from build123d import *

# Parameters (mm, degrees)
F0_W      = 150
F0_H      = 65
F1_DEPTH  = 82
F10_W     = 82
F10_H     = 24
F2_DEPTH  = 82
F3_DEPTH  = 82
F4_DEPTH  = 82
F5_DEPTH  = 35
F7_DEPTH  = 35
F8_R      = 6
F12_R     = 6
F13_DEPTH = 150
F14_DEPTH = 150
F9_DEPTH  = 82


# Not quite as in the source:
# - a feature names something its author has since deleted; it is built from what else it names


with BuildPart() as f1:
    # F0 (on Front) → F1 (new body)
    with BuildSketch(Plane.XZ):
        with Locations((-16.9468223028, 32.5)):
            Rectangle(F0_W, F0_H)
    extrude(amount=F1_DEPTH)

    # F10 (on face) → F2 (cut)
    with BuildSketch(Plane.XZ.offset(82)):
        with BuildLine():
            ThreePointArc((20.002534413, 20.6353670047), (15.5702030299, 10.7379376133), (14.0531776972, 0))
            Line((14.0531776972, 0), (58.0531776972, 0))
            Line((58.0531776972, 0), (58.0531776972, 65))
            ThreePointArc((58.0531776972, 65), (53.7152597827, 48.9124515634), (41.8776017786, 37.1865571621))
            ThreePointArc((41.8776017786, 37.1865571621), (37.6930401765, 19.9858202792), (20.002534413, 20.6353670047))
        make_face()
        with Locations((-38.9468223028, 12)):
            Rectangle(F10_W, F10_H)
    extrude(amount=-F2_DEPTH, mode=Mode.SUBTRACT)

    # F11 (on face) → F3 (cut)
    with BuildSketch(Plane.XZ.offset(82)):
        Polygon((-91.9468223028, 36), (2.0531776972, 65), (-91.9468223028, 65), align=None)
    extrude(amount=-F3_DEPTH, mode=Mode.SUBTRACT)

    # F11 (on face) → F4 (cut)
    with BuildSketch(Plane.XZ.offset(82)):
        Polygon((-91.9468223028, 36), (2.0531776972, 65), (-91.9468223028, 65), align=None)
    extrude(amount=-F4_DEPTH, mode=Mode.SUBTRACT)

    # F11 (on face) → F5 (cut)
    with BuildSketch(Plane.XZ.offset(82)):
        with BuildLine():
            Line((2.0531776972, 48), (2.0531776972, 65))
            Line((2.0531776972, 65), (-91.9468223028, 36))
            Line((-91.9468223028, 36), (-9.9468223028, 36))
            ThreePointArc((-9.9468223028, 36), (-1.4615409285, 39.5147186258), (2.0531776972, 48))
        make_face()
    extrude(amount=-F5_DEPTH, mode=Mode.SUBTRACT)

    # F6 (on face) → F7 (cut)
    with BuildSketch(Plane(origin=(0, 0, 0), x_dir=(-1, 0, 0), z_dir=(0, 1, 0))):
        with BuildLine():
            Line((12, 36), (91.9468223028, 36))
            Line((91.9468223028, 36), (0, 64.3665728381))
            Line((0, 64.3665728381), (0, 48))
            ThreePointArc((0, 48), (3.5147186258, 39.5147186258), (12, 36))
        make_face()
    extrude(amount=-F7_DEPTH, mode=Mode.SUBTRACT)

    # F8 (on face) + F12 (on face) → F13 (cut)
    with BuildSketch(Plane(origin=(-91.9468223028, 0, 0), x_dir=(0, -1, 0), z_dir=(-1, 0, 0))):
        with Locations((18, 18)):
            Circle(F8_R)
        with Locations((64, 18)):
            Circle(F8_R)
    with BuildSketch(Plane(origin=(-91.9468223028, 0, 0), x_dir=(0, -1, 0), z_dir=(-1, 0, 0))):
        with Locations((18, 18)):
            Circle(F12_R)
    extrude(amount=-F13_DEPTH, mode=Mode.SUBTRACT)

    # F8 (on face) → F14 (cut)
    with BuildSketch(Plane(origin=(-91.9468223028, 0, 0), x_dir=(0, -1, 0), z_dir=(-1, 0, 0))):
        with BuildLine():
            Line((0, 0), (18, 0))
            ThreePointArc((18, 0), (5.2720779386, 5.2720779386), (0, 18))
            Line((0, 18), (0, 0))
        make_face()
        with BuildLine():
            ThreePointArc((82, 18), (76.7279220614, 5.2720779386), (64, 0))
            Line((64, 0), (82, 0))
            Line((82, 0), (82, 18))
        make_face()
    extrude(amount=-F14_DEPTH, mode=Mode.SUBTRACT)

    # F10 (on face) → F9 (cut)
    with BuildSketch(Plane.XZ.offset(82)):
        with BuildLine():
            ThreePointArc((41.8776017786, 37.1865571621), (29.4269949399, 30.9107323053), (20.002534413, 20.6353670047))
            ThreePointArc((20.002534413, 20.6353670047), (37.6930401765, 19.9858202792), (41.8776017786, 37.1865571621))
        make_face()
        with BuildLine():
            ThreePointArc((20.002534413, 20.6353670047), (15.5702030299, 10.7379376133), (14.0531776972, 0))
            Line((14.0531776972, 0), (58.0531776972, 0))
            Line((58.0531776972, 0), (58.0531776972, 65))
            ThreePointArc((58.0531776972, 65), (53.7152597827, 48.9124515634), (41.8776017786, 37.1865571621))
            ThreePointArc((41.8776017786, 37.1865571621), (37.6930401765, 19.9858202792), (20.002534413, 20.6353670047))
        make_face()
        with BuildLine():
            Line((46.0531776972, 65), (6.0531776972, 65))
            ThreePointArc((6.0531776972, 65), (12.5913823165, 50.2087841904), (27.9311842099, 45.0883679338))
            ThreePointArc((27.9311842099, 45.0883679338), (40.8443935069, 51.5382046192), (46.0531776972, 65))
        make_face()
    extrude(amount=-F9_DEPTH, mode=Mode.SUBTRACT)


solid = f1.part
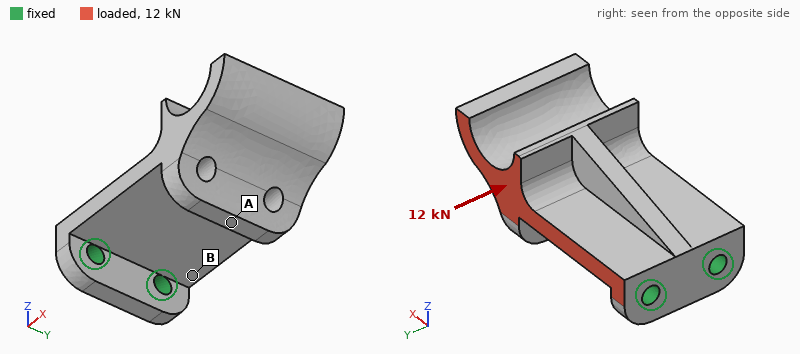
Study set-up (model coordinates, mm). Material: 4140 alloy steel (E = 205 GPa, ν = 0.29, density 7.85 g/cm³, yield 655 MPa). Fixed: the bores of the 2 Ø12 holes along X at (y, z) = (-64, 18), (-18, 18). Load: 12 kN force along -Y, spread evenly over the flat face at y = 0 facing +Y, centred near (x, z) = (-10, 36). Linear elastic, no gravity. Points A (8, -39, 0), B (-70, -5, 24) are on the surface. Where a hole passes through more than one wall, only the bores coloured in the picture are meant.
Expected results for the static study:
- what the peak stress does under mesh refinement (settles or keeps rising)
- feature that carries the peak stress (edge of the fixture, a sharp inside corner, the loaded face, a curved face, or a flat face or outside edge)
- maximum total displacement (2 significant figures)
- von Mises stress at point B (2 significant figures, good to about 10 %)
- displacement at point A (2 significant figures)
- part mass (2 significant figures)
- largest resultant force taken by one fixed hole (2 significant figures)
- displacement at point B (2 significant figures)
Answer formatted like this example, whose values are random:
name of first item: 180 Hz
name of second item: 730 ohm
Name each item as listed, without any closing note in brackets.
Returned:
what the peak stress does under mesh refinement: keeps rising
feature that carries the peak stress: edge of the fixture
maximum total displacement: 0.11 mm
von Mises stress at point B: 78 MPa
displacement at point A: 0.047 mm
part mass: 2.0 kg
largest resultant force taken by one fixed hole: 18 kN
displacement at point B: 0.017 mm
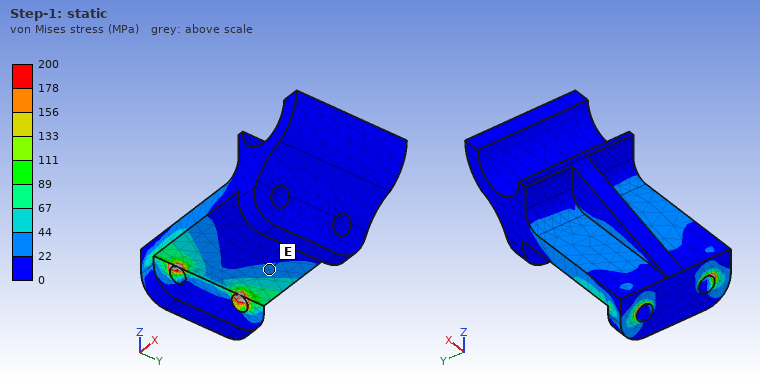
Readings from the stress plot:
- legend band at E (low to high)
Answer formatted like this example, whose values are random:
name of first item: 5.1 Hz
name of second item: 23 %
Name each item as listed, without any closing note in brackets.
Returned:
legend band at E: 22 to 44 MPa
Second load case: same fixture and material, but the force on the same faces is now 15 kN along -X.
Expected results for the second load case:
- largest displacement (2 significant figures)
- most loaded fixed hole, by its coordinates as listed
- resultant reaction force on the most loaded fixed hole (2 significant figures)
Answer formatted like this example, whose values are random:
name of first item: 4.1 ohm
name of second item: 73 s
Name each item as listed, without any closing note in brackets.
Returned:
largest displacement: 0.30 mm
most loaded fixed hole, by its coordinates as listed: (-18, 18)
resultant reaction force on the most loaded fixed hole: 19 kN
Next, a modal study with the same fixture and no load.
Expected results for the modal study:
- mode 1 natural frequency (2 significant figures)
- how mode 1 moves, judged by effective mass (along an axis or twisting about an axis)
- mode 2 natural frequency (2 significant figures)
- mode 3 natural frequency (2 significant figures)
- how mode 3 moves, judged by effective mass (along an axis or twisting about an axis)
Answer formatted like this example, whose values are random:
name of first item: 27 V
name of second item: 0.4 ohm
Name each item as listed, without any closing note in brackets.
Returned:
mode 1 natural frequency: 400 Hz
how mode 1 moves, judged by effective mass: along Z
mode 2 natural frequency: 1400 Hz
mode 3 natural frequency: 1600 Hz
how mode 3 moves, judged by effective mass: along Y
